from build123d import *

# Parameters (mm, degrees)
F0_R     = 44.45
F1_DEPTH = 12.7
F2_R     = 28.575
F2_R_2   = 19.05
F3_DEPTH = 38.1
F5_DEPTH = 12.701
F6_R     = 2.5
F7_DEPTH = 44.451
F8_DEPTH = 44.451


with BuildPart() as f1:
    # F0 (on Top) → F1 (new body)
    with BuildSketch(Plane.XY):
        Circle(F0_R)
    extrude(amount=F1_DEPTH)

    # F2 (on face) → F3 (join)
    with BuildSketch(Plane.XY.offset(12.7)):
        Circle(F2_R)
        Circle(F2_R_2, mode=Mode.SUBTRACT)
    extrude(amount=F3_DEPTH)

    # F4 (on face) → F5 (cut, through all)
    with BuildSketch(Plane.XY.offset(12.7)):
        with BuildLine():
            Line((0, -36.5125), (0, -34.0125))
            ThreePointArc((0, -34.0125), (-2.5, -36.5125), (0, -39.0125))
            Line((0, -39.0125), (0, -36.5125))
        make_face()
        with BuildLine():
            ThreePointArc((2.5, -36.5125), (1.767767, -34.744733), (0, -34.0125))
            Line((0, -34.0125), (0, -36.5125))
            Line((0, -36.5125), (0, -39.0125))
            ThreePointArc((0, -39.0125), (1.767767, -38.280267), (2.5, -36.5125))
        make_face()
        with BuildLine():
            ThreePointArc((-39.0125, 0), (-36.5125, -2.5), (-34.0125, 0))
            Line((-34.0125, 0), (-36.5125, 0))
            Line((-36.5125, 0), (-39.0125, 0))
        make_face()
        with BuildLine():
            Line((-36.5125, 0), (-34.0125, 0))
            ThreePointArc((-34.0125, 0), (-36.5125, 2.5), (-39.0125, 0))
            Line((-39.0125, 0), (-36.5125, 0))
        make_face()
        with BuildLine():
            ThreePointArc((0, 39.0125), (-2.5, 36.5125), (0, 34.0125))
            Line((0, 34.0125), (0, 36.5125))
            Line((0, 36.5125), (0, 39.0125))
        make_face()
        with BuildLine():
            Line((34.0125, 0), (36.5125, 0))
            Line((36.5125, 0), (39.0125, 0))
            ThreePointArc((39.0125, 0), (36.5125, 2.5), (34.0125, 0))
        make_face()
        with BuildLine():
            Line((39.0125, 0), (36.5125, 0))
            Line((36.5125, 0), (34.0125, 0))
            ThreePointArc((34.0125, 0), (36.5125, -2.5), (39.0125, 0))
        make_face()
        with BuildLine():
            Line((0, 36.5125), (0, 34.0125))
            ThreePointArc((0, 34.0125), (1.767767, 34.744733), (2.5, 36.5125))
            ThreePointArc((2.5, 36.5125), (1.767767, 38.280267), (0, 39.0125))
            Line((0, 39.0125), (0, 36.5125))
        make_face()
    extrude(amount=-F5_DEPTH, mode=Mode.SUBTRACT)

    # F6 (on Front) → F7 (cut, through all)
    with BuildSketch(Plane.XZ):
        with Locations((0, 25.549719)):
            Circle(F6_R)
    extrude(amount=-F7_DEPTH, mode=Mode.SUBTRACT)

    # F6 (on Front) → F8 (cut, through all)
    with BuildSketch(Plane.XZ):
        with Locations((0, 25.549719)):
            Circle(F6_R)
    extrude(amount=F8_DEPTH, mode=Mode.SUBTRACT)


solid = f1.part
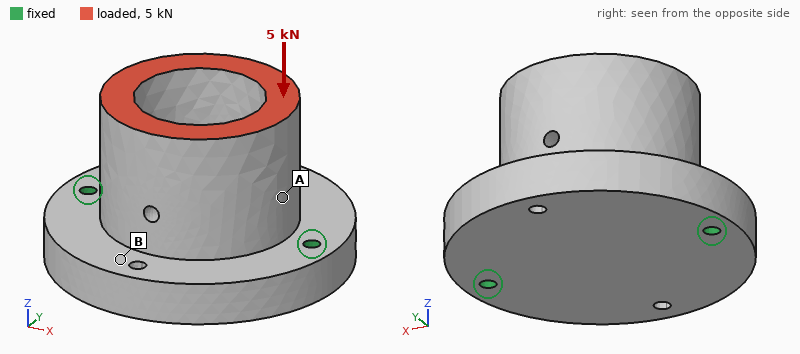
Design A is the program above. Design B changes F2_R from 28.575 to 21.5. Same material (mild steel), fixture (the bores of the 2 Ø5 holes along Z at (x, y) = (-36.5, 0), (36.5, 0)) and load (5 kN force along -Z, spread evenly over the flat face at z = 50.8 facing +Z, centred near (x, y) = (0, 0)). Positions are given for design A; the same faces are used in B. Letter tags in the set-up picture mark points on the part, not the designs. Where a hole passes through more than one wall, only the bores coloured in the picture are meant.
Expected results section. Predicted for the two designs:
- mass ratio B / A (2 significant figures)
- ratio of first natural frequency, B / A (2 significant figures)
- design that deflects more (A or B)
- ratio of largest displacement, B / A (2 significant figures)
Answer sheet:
0.68
1.3
B
2.9
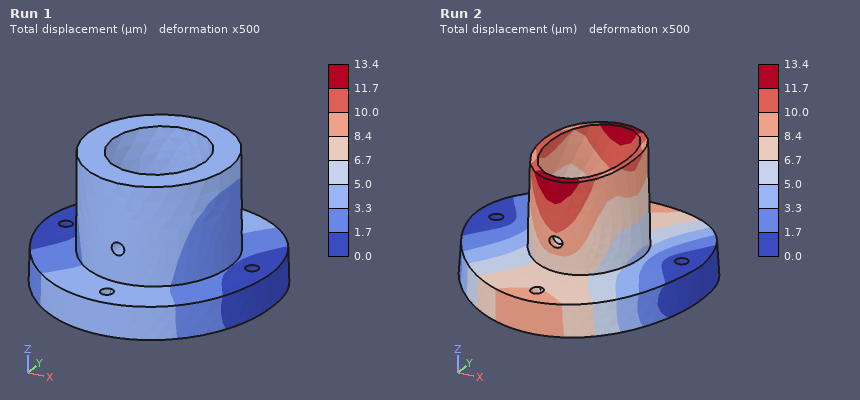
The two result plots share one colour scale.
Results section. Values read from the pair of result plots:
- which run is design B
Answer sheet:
Run 2
